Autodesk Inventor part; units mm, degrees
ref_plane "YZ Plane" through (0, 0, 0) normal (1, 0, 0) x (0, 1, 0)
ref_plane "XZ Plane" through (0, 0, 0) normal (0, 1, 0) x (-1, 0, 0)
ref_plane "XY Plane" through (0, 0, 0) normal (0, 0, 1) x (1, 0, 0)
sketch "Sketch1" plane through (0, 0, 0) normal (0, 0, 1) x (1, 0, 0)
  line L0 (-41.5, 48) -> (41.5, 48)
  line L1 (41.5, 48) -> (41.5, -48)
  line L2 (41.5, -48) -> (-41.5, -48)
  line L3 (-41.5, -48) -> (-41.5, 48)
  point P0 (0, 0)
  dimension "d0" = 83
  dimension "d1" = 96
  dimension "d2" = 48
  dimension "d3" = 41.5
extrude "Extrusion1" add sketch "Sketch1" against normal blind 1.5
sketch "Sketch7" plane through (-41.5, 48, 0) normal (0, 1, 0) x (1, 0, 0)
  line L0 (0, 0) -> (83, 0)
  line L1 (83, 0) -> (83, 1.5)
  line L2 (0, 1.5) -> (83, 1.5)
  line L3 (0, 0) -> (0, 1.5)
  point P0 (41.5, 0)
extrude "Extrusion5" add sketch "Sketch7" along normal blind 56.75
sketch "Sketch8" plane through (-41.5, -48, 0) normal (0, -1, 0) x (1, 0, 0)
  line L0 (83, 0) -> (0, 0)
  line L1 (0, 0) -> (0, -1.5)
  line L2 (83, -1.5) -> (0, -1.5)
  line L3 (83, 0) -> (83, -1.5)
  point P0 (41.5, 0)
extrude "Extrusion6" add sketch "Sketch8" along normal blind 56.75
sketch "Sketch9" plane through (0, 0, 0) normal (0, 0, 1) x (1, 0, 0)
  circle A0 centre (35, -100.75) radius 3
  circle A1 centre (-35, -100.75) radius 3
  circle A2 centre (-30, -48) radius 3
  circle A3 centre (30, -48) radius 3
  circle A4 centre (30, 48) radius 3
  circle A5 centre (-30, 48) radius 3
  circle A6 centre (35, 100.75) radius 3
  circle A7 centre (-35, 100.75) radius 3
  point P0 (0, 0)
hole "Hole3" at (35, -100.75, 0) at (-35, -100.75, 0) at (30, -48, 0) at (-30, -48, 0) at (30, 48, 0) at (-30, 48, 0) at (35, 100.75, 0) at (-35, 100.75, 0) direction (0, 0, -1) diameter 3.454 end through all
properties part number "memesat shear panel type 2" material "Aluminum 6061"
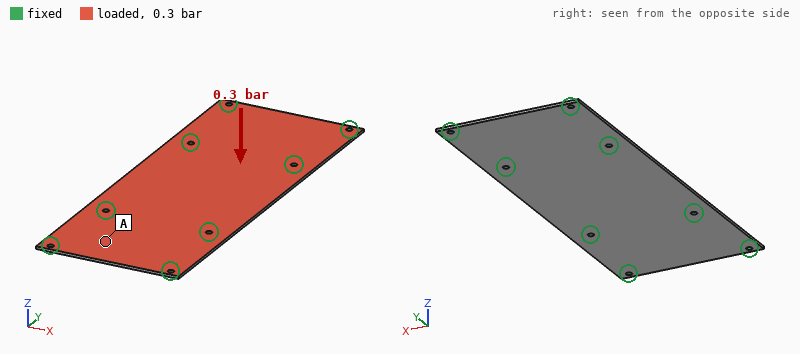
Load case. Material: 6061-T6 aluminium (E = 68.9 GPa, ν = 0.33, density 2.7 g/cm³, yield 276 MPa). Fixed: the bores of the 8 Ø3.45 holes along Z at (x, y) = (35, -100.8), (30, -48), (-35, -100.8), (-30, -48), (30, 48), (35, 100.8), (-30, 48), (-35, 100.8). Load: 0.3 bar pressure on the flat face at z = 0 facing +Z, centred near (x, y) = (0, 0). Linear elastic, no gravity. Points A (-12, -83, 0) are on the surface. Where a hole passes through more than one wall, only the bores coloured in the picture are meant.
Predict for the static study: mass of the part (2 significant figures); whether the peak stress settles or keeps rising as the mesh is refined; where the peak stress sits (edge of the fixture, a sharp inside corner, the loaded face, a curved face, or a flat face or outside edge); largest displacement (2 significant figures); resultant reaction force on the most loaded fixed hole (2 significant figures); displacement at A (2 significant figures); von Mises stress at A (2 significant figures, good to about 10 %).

70 g
keeps rising
edge of the fixture
0.41 mm
98 N
0.090 mm
10 MPa
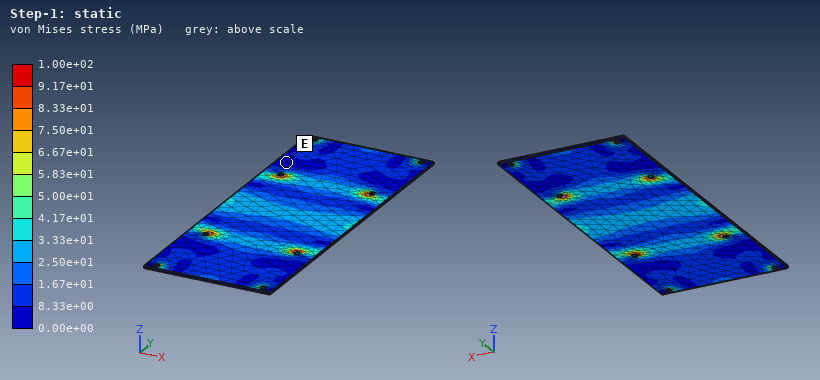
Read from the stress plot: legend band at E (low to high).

0.00e+00 to 8.33e+00 MPa
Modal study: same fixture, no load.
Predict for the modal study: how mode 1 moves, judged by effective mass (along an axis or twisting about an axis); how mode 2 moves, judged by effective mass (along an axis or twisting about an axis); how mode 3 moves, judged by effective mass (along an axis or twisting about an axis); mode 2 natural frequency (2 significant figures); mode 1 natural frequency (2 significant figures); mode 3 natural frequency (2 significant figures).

along Z
twisting about Y
along Z
1100 Hz
770 Hz
1500 Hz
